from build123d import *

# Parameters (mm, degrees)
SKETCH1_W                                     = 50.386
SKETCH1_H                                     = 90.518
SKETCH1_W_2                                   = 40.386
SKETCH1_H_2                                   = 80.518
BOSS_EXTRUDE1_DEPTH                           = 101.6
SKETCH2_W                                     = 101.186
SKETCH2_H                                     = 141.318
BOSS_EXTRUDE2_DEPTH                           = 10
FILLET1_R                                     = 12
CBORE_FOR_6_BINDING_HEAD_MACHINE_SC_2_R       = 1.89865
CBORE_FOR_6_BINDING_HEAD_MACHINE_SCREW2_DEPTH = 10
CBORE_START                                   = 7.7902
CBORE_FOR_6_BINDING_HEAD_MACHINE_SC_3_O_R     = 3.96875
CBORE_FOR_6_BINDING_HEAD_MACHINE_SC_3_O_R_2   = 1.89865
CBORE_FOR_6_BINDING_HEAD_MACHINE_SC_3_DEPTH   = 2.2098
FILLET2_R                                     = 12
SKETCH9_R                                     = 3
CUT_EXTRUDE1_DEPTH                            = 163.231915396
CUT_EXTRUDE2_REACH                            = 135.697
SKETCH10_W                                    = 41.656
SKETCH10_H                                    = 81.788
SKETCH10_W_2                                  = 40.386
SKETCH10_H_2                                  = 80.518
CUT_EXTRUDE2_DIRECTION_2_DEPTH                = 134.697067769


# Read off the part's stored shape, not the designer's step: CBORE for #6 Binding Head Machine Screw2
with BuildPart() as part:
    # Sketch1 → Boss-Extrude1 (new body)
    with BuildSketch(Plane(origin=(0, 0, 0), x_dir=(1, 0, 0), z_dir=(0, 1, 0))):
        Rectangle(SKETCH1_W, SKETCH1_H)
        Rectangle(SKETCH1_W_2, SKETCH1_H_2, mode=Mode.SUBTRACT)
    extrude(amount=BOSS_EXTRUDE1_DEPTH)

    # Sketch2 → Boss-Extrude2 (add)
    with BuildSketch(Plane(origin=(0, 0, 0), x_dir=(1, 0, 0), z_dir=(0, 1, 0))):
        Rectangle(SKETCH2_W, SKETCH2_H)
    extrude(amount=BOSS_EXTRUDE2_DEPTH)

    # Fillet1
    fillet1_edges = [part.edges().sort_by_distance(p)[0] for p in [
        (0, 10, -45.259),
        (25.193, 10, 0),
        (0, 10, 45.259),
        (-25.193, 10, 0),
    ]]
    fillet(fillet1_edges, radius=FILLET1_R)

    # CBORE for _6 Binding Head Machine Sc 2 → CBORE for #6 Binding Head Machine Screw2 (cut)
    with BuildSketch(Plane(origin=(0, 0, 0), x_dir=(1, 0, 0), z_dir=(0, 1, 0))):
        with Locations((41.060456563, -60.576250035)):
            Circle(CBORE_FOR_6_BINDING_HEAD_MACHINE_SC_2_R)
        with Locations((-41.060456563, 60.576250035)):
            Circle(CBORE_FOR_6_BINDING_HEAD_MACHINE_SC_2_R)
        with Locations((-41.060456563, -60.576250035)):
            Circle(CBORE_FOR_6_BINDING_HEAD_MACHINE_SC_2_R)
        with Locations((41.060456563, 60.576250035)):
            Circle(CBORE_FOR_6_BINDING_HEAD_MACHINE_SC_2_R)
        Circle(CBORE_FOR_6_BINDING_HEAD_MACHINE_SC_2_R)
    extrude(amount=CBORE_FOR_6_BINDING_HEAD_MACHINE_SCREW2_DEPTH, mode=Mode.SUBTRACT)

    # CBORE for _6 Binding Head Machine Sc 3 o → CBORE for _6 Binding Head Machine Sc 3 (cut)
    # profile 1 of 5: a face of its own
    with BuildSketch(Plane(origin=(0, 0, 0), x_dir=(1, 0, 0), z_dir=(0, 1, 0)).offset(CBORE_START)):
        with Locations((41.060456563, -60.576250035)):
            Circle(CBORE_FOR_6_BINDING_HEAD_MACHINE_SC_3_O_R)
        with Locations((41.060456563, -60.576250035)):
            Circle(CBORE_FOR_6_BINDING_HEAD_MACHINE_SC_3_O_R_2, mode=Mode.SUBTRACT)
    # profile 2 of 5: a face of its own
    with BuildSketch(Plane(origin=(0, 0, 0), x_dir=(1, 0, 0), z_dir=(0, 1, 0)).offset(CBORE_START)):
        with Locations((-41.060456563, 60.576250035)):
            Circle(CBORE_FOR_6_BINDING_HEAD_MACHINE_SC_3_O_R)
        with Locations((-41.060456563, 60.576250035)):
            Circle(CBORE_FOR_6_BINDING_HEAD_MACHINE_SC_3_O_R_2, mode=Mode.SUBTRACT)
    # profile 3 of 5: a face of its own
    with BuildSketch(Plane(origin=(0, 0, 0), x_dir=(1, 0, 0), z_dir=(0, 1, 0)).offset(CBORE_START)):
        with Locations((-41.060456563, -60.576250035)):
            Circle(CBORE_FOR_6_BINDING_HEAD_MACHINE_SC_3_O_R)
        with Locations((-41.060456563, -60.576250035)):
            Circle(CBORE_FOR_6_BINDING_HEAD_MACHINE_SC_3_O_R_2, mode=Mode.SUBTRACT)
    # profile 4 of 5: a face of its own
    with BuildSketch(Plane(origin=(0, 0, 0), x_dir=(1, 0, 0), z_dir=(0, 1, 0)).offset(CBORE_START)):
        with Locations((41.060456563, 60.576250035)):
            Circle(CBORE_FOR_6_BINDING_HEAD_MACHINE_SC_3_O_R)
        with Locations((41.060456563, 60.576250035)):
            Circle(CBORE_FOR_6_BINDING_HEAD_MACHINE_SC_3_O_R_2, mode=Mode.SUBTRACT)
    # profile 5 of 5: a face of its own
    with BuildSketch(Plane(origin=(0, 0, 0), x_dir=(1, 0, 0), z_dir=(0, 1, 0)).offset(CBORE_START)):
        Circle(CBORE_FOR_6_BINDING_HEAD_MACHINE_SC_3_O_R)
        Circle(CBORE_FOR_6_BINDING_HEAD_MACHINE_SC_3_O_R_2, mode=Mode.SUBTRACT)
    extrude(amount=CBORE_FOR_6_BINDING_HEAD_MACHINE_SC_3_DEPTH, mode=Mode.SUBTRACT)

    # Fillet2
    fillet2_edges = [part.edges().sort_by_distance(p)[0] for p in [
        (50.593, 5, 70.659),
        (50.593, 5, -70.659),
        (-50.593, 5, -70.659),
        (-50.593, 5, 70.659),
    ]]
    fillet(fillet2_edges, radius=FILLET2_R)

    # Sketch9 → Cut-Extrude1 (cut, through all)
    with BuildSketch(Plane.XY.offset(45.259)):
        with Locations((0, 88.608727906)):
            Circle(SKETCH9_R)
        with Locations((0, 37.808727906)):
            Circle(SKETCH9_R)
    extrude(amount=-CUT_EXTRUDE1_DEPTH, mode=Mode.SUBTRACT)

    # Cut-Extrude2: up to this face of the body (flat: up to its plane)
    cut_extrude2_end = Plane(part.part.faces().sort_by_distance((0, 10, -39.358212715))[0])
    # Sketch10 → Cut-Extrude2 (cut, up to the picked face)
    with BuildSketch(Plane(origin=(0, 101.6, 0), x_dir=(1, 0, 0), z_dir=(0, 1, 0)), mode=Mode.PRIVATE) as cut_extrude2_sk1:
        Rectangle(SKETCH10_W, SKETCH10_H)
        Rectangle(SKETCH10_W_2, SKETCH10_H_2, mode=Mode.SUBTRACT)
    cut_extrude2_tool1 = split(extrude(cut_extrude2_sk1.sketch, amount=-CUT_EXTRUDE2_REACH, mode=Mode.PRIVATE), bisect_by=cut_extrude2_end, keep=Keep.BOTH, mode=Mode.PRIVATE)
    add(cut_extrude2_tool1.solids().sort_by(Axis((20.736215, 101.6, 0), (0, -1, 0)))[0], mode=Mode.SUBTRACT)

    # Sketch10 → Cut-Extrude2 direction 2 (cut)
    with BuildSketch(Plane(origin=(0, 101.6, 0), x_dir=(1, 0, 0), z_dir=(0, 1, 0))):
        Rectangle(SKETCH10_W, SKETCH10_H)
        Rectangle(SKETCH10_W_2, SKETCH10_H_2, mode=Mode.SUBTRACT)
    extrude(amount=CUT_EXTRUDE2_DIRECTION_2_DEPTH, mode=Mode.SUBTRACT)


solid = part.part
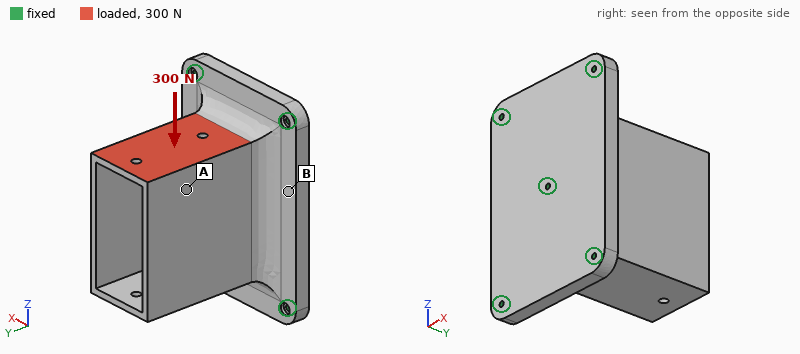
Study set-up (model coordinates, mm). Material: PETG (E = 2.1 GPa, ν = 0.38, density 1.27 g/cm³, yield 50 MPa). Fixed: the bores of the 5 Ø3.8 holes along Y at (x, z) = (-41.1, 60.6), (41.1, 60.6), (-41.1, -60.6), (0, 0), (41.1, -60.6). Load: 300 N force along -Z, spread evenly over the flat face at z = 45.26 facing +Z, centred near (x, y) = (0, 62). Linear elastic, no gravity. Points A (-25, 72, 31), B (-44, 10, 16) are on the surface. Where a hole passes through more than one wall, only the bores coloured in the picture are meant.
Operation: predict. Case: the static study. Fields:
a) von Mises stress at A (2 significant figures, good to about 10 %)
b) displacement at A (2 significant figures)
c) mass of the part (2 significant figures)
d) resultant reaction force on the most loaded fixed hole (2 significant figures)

1.0 MPa
0.10 mm
320 g
110 N
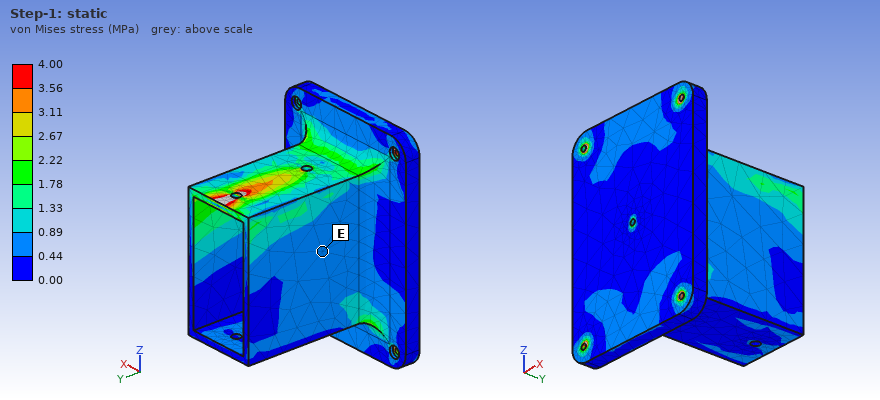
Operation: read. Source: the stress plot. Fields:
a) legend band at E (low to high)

0.44 to 0.89 MPa
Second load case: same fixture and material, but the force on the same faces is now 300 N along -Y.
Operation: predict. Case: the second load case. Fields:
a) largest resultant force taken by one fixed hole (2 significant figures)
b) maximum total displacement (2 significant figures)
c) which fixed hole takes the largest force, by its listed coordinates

130 N
0.12 mm
(0, 0)
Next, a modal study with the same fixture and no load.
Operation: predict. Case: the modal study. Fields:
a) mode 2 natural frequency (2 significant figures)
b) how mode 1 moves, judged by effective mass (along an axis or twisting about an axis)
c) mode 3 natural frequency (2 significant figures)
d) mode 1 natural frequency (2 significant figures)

590 Hz
along X
780 Hz
500 Hz
